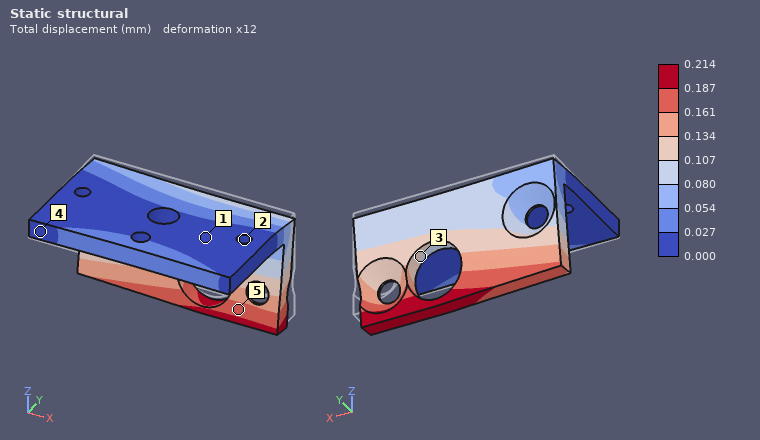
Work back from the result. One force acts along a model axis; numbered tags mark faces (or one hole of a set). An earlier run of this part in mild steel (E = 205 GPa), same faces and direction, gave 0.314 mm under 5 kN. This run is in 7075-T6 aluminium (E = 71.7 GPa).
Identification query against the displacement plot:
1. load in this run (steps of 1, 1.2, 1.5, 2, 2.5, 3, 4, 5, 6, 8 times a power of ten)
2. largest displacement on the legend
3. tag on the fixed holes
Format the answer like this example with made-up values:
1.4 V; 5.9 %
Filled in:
1.2 kN; 0.214 mm; 2
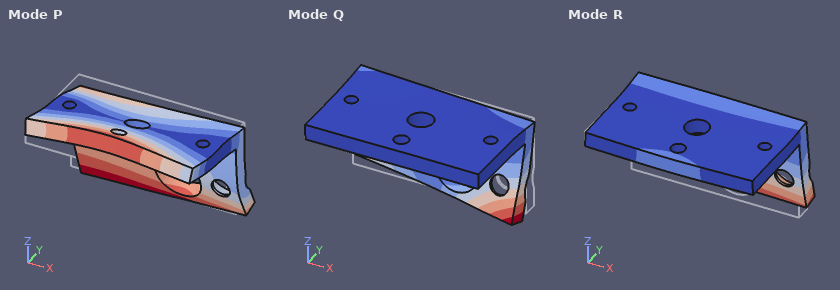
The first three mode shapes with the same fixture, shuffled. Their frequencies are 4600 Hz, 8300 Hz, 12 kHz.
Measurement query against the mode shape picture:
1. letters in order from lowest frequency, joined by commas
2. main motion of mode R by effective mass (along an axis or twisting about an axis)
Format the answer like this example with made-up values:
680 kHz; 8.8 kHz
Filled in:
R, Q, P; along Y
